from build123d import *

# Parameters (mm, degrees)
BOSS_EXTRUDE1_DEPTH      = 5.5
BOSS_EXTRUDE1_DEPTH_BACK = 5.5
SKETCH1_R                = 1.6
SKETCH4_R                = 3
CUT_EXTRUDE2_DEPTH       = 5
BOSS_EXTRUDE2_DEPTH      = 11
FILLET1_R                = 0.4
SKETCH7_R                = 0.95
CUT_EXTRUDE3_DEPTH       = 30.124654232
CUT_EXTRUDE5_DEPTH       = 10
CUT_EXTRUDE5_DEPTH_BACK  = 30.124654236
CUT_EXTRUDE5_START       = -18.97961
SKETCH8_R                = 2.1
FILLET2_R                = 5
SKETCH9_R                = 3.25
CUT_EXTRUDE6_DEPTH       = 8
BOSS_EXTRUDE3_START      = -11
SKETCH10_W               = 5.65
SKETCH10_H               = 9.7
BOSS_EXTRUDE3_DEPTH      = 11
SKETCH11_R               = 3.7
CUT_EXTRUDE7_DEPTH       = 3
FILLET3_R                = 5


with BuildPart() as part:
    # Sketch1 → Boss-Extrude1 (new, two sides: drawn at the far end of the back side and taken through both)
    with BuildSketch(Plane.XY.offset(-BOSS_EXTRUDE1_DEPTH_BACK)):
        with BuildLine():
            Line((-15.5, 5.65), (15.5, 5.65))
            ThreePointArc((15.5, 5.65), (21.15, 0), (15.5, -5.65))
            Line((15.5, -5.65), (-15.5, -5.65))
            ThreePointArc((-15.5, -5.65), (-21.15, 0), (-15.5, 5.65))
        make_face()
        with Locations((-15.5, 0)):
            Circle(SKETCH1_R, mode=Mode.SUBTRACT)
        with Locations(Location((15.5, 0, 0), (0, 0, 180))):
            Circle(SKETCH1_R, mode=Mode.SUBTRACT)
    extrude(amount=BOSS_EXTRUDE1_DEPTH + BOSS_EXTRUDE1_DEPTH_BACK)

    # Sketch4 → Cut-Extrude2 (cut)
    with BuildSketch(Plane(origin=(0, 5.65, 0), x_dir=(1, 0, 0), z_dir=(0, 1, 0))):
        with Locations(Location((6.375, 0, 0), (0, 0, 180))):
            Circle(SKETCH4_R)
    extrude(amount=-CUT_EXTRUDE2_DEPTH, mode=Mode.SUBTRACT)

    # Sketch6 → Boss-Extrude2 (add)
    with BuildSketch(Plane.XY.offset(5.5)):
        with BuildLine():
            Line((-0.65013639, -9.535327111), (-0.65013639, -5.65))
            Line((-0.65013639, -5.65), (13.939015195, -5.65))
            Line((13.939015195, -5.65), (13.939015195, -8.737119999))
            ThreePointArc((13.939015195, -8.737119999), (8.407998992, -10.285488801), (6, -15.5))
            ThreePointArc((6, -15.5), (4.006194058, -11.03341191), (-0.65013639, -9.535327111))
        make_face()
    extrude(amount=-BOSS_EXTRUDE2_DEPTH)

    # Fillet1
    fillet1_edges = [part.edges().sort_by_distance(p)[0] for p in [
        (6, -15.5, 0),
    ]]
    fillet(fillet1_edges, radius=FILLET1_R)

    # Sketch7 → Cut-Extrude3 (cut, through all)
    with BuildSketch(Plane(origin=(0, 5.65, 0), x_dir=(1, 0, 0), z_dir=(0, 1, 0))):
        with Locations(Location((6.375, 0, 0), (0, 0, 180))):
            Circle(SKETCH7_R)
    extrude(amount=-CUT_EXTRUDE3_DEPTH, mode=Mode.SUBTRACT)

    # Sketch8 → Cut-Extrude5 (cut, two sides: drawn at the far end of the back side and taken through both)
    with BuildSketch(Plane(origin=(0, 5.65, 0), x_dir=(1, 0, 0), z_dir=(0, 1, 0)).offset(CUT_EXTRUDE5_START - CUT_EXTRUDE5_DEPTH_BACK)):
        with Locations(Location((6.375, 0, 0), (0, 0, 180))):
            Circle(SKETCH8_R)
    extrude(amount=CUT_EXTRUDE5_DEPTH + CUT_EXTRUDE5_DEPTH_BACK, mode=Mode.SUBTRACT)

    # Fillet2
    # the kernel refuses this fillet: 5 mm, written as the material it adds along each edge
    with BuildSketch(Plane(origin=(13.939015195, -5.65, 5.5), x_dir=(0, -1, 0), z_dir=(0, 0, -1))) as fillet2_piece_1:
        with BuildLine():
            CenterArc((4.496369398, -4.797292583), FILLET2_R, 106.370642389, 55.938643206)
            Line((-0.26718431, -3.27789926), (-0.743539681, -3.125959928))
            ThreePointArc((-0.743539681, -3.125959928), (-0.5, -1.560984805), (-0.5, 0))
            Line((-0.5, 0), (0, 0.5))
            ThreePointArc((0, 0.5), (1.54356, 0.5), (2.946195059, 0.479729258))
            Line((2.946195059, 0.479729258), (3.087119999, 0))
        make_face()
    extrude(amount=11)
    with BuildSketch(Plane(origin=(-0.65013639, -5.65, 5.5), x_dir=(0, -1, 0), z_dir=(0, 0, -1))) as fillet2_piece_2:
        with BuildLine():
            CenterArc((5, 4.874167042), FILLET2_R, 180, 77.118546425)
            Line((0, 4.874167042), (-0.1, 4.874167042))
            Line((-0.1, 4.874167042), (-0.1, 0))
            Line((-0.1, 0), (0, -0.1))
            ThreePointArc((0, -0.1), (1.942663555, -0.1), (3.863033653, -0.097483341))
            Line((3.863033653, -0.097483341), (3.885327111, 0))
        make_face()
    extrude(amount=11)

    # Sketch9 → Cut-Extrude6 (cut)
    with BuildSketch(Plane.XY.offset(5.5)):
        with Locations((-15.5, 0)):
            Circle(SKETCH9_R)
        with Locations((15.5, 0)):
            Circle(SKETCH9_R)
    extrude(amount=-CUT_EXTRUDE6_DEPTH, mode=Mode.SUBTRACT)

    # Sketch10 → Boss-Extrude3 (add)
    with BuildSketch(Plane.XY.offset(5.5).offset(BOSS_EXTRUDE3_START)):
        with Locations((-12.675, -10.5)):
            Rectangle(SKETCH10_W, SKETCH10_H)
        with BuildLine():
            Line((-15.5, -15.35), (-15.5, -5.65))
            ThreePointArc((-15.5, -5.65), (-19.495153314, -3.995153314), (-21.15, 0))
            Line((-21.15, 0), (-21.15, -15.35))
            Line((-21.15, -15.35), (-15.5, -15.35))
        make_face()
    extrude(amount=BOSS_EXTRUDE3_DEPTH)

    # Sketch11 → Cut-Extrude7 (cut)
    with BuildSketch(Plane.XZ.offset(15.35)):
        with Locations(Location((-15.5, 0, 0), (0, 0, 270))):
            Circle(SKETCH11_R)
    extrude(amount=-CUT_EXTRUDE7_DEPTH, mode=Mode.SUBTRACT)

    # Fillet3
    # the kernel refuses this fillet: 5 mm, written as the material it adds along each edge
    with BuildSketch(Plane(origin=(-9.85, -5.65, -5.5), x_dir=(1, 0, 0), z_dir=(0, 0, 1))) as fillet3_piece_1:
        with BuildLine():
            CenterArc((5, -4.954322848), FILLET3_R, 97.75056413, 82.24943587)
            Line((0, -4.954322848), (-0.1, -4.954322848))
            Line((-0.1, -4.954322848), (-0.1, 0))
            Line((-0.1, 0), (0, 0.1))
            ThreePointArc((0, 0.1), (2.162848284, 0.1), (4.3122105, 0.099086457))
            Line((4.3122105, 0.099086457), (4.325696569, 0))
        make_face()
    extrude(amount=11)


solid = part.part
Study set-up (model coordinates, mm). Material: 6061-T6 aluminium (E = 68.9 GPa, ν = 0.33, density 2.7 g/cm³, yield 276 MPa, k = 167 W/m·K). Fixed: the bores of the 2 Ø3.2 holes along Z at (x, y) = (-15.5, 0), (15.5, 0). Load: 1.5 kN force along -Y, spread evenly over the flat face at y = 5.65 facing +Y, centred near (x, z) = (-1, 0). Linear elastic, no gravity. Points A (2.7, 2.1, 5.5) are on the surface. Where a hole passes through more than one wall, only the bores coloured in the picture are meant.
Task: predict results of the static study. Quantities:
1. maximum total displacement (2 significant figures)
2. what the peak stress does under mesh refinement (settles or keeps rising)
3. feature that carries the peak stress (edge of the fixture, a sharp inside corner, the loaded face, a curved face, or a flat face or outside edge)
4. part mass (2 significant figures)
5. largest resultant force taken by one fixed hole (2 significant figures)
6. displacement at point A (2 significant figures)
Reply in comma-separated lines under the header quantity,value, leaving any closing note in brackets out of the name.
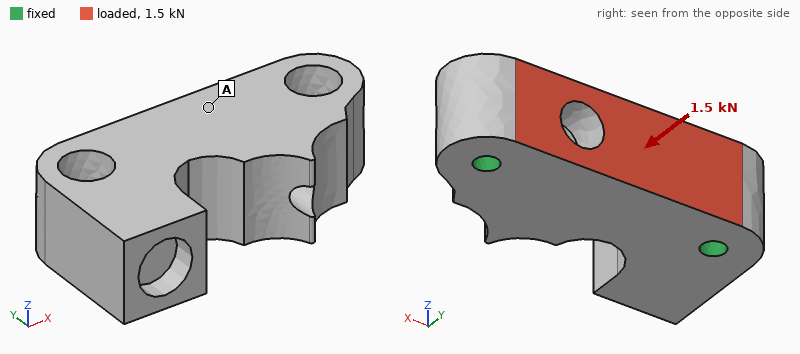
quantity,value
maximum total displacement,35 µm
what the peak stress does under mesh refinement,keeps rising
feature that carries the peak stress,edge of the fixture
part mass,17 g
largest resultant force taken by one fixed hole,780 N
displacement at point A,24 µm
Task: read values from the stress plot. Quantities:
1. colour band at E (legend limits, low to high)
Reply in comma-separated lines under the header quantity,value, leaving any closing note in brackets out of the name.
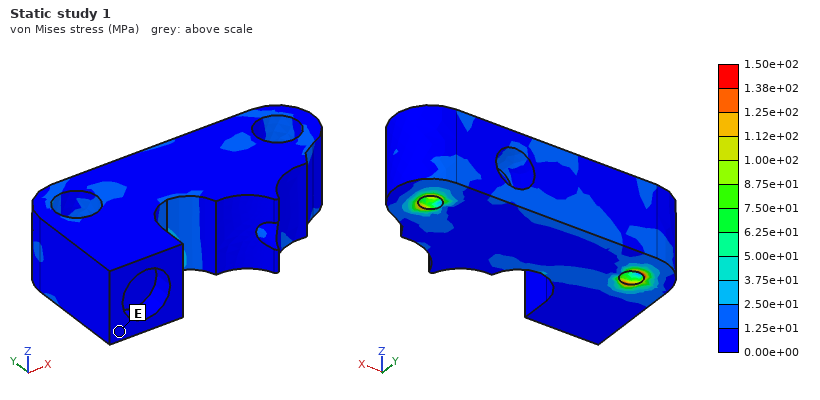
quantity,value
colour band at E,0.00e+00 to 1.25e+01 MPa
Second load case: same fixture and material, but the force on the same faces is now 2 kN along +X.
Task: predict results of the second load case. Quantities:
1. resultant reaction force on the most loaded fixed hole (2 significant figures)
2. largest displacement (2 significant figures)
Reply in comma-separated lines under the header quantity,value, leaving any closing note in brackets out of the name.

quantity,value
resultant reaction force on the most loaded fixed hole,1.1 kN
largest displacement,7.2 µm
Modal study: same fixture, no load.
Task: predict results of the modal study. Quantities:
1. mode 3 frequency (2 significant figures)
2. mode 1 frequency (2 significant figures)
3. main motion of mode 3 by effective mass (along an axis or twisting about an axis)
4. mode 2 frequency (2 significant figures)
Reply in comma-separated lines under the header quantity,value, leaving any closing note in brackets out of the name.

quantity,value
mode 3 frequency,21 kHz
mode 1 frequency,9000 Hz
main motion of mode 3 by effective mass,along Z
mode 2 frequency,19 kHz
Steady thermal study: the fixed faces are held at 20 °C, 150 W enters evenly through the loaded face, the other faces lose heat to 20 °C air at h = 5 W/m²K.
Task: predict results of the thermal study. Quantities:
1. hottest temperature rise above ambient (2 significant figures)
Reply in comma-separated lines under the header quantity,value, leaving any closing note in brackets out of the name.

quantity,value
hottest temperature rise above ambient,66 K
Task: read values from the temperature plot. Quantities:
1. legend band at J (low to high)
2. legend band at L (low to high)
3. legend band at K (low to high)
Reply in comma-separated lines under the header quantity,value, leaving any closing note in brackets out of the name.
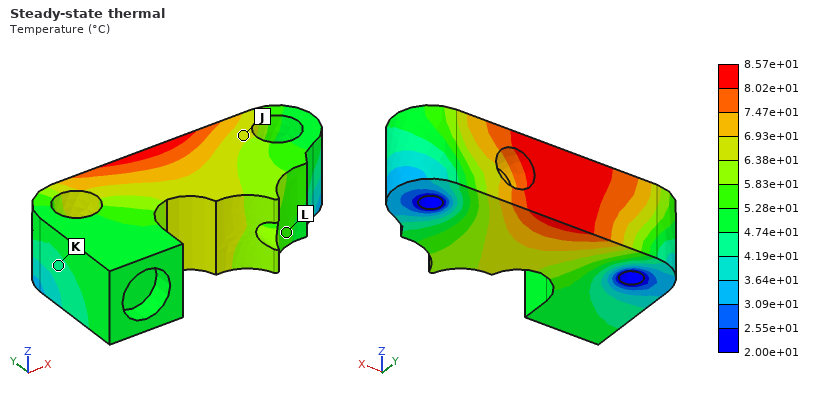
quantity,value
legend band at J,6.38e+01 to 6.93e+01 °C
legend band at L,5.28e+01 to 5.83e+01 °C
legend band at K,4.19e+01 to 4.74e+01 °C
